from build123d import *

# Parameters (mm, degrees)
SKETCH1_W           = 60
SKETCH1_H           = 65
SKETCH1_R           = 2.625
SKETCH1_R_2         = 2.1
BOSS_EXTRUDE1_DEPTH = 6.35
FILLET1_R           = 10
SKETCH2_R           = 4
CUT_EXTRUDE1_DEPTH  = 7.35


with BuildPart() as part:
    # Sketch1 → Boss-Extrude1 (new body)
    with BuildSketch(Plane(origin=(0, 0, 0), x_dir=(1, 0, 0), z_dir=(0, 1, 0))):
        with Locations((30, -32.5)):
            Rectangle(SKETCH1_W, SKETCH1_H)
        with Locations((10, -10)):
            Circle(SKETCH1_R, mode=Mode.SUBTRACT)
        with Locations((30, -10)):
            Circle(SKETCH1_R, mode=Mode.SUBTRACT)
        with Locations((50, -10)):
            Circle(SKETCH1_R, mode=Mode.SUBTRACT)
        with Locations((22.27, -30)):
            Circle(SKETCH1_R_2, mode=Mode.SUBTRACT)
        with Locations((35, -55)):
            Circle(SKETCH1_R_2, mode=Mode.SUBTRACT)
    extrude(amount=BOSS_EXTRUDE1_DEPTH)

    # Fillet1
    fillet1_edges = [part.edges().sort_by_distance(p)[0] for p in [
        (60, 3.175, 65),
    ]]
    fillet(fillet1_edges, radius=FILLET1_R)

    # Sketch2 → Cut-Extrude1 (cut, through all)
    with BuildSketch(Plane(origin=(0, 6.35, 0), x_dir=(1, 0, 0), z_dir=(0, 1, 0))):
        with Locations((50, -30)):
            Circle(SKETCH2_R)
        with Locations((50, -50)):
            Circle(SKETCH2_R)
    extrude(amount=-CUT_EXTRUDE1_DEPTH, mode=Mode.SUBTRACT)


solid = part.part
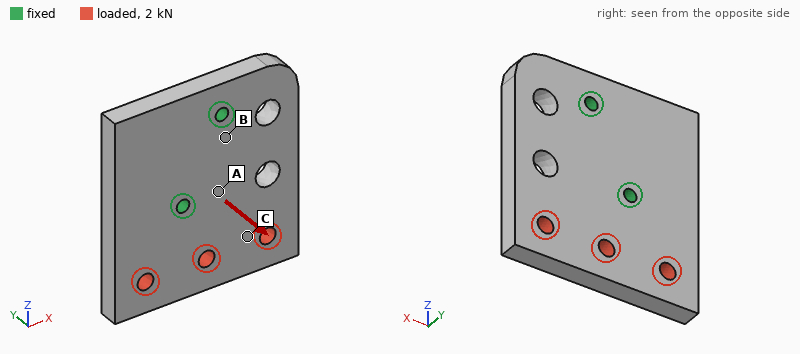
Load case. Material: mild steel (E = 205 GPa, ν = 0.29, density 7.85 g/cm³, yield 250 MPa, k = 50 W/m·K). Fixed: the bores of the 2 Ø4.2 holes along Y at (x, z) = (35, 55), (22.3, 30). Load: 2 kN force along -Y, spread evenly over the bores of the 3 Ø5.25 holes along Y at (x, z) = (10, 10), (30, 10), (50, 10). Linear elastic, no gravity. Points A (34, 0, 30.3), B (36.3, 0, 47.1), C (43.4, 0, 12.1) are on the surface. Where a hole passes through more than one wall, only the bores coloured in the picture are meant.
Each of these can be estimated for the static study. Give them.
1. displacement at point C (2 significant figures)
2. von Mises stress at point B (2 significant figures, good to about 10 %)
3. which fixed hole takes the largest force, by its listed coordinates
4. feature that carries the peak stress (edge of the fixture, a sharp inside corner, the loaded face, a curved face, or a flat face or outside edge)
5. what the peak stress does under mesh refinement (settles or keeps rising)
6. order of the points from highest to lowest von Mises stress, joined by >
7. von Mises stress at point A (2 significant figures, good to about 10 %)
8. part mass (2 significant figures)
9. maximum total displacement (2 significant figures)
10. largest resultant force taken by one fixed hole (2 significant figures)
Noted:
0.062 mm
39 MPa
(22.3, 30)
edge of the fixture
keeps rising
A > B > C
78 MPa
180 g
0.12 mm
2.4 kN
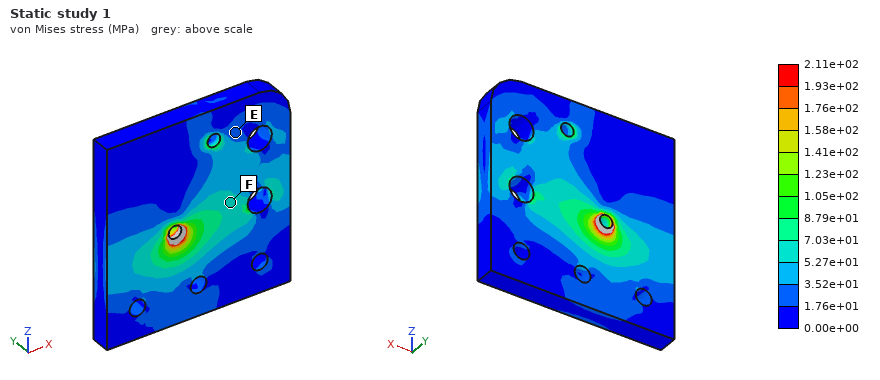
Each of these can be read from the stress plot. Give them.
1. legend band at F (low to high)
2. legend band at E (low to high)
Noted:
5.27e+01 to 7.03e+01 MPa
1.76e+01 to 3.52e+01 MPa
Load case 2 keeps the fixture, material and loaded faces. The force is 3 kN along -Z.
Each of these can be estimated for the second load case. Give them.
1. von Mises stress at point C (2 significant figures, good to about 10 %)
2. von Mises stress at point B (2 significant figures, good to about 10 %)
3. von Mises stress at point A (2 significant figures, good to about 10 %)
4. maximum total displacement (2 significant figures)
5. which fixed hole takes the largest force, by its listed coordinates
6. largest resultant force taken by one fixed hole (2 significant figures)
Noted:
8.0 MPa
12 MPa
9.2 MPa
3.2 µm
(22.3, 30)
1.9 kN
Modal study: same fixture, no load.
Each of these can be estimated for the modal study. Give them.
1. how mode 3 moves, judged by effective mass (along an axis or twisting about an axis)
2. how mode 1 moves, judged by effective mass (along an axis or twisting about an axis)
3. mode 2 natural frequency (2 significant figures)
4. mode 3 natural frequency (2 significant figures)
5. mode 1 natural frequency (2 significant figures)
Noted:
along Y
along Y
5200 Hz
6200 Hz
3200 Hz
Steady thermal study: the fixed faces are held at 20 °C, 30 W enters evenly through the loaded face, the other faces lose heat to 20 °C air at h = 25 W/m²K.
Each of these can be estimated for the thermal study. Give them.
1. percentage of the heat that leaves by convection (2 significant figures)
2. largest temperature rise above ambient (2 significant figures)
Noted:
16 %
53 K
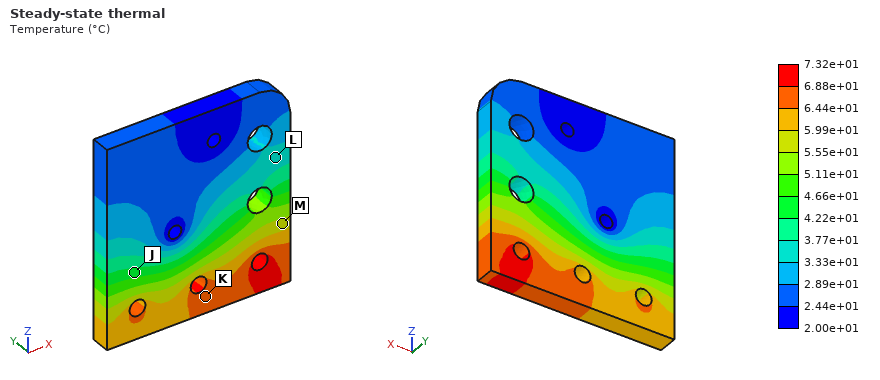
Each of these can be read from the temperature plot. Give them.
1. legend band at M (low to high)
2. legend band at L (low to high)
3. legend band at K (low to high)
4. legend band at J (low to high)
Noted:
5.55e+01 to 5.99e+01 °C
3.33e+01 to 3.77e+01 °C
6.44e+01 to 6.88e+01 °C
4.22e+01 to 4.66e+01 °C
